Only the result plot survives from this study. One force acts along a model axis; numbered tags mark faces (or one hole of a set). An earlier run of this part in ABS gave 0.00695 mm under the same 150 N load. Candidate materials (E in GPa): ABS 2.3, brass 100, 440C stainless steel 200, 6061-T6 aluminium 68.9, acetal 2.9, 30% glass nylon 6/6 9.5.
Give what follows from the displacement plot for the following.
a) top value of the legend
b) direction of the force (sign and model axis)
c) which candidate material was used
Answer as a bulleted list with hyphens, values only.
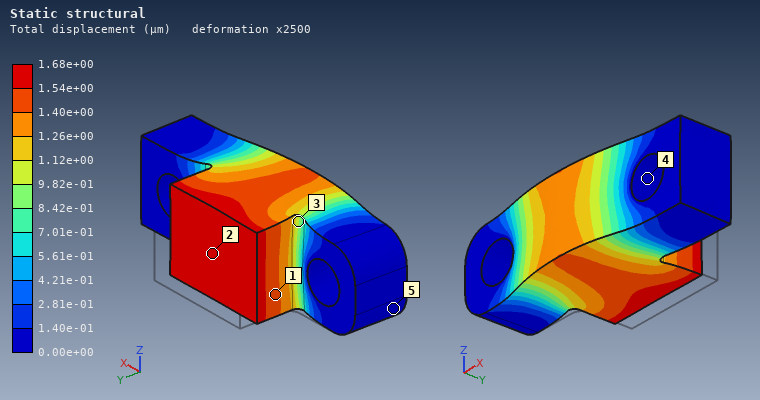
- 1.68e+00 µm
- -Y
- 30% glass nylon 6/6
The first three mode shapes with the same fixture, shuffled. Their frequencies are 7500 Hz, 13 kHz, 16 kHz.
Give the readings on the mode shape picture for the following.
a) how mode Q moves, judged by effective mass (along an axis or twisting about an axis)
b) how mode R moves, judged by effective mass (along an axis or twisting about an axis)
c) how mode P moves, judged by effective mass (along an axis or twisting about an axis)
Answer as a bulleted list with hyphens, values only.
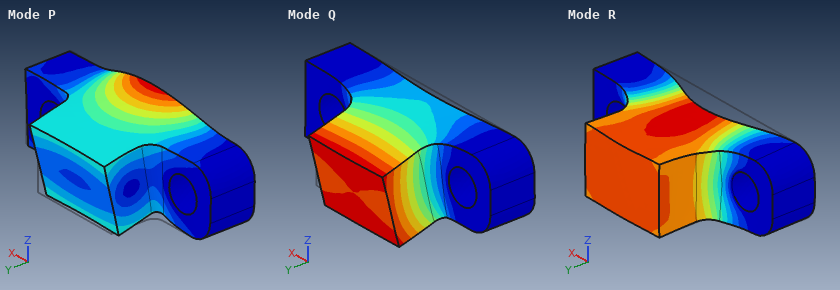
- along Z
- along Y
- along Z
